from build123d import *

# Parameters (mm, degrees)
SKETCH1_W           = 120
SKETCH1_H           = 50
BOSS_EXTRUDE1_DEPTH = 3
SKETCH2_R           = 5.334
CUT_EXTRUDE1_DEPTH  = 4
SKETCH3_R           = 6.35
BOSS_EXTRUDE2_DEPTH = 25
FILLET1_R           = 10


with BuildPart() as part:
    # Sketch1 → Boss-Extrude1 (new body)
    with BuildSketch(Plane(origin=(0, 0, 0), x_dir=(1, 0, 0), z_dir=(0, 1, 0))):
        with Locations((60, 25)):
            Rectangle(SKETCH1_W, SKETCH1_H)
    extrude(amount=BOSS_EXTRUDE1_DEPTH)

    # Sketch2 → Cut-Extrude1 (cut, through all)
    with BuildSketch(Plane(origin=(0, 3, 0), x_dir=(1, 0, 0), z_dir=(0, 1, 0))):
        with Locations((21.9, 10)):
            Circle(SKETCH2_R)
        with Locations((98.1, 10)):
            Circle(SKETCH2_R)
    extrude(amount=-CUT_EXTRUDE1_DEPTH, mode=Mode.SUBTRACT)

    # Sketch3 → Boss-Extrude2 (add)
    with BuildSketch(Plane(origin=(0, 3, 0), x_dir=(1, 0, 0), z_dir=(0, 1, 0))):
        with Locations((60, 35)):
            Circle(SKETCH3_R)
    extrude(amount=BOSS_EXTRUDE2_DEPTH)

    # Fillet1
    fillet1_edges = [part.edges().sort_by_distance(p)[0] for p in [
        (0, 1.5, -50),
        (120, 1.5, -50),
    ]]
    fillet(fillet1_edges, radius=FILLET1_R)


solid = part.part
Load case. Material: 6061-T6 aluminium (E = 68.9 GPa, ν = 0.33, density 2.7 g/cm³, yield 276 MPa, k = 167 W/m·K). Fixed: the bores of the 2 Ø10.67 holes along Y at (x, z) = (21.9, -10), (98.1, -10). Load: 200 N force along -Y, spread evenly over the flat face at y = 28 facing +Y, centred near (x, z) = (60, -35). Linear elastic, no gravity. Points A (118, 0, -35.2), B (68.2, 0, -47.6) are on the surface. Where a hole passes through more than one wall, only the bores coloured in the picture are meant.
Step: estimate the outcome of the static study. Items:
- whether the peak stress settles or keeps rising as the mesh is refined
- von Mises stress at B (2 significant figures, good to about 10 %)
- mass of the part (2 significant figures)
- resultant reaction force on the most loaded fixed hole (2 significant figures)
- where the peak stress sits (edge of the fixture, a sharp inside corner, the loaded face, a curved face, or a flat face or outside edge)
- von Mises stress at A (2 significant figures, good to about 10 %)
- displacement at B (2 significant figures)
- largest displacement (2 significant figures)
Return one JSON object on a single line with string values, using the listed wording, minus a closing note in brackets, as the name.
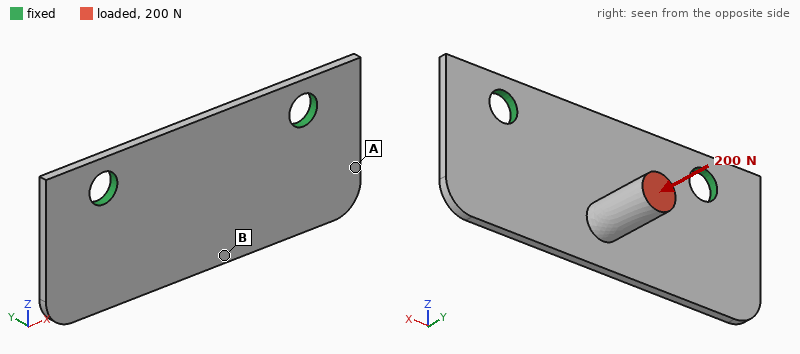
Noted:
{"whether the peak stress settles or keeps rising as the mesh is refined": "keeps rising", "von Mises stress at B": "23 MPa", "mass of the part": "55 g", "resultant reaction force on the most loaded fixed hole": "100 N", "where the peak stress sits": "edge of the fixture", "von Mises stress at A": "11 MPa", "displacement at B": "0.20 mm", "largest displacement": "0.22 mm"}
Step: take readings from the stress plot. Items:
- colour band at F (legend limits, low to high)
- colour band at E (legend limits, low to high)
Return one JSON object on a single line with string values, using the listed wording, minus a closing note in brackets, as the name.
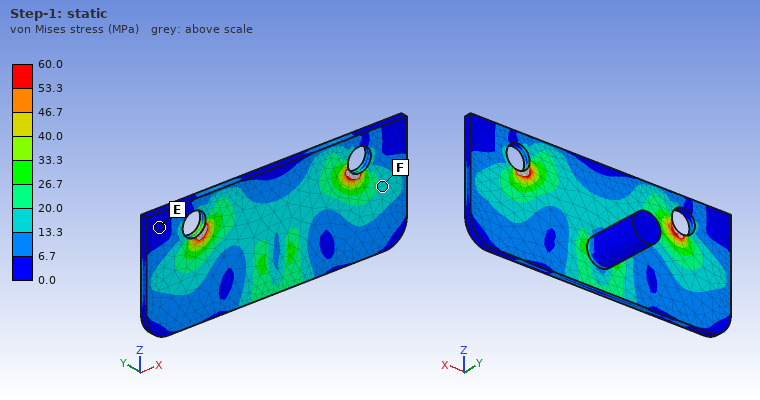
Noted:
{"colour band at F": "13.3 to 20.0 MPa", "colour band at E": "0.0 to 6.7 MPa"}
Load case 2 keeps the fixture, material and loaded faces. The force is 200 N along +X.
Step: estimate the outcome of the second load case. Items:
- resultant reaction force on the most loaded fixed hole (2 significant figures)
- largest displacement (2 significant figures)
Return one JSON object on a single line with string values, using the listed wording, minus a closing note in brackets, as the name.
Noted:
{"resultant reaction force on the most loaded fixed hole": "150 N", "largest displacement": "0.14 mm"}
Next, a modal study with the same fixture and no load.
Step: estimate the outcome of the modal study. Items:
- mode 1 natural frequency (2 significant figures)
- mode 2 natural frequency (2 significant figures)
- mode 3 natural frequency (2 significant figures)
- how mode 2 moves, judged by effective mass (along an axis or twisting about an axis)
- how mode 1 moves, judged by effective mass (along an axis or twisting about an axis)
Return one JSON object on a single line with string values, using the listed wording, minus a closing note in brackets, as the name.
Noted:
{"mode 1 natural frequency": "1100 Hz", "mode 2 natural frequency": "2100 Hz", "mode 3 natural frequency": "2500 Hz", "how mode 2 moves, judged by effective mass": "twisting about Z", "how mode 1 moves, judged by effective mass": "along Y"}
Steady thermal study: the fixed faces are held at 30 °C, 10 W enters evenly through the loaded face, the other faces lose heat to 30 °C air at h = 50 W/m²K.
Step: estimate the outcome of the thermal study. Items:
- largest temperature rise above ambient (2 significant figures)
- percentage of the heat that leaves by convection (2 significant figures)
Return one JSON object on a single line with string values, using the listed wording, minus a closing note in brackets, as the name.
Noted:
{"largest temperature rise above ambient": "21 K", "percentage of the heat that leaves by convection": "27 %"}
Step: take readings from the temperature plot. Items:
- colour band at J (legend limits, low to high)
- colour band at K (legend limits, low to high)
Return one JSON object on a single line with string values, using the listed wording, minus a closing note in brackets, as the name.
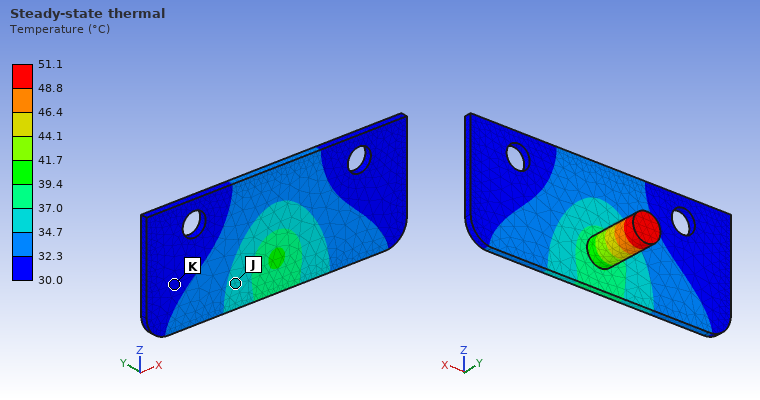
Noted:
{"colour band at J": "34.7 to 37.0 °C", "colour band at K": "30.0 to 32.3 °C"}
